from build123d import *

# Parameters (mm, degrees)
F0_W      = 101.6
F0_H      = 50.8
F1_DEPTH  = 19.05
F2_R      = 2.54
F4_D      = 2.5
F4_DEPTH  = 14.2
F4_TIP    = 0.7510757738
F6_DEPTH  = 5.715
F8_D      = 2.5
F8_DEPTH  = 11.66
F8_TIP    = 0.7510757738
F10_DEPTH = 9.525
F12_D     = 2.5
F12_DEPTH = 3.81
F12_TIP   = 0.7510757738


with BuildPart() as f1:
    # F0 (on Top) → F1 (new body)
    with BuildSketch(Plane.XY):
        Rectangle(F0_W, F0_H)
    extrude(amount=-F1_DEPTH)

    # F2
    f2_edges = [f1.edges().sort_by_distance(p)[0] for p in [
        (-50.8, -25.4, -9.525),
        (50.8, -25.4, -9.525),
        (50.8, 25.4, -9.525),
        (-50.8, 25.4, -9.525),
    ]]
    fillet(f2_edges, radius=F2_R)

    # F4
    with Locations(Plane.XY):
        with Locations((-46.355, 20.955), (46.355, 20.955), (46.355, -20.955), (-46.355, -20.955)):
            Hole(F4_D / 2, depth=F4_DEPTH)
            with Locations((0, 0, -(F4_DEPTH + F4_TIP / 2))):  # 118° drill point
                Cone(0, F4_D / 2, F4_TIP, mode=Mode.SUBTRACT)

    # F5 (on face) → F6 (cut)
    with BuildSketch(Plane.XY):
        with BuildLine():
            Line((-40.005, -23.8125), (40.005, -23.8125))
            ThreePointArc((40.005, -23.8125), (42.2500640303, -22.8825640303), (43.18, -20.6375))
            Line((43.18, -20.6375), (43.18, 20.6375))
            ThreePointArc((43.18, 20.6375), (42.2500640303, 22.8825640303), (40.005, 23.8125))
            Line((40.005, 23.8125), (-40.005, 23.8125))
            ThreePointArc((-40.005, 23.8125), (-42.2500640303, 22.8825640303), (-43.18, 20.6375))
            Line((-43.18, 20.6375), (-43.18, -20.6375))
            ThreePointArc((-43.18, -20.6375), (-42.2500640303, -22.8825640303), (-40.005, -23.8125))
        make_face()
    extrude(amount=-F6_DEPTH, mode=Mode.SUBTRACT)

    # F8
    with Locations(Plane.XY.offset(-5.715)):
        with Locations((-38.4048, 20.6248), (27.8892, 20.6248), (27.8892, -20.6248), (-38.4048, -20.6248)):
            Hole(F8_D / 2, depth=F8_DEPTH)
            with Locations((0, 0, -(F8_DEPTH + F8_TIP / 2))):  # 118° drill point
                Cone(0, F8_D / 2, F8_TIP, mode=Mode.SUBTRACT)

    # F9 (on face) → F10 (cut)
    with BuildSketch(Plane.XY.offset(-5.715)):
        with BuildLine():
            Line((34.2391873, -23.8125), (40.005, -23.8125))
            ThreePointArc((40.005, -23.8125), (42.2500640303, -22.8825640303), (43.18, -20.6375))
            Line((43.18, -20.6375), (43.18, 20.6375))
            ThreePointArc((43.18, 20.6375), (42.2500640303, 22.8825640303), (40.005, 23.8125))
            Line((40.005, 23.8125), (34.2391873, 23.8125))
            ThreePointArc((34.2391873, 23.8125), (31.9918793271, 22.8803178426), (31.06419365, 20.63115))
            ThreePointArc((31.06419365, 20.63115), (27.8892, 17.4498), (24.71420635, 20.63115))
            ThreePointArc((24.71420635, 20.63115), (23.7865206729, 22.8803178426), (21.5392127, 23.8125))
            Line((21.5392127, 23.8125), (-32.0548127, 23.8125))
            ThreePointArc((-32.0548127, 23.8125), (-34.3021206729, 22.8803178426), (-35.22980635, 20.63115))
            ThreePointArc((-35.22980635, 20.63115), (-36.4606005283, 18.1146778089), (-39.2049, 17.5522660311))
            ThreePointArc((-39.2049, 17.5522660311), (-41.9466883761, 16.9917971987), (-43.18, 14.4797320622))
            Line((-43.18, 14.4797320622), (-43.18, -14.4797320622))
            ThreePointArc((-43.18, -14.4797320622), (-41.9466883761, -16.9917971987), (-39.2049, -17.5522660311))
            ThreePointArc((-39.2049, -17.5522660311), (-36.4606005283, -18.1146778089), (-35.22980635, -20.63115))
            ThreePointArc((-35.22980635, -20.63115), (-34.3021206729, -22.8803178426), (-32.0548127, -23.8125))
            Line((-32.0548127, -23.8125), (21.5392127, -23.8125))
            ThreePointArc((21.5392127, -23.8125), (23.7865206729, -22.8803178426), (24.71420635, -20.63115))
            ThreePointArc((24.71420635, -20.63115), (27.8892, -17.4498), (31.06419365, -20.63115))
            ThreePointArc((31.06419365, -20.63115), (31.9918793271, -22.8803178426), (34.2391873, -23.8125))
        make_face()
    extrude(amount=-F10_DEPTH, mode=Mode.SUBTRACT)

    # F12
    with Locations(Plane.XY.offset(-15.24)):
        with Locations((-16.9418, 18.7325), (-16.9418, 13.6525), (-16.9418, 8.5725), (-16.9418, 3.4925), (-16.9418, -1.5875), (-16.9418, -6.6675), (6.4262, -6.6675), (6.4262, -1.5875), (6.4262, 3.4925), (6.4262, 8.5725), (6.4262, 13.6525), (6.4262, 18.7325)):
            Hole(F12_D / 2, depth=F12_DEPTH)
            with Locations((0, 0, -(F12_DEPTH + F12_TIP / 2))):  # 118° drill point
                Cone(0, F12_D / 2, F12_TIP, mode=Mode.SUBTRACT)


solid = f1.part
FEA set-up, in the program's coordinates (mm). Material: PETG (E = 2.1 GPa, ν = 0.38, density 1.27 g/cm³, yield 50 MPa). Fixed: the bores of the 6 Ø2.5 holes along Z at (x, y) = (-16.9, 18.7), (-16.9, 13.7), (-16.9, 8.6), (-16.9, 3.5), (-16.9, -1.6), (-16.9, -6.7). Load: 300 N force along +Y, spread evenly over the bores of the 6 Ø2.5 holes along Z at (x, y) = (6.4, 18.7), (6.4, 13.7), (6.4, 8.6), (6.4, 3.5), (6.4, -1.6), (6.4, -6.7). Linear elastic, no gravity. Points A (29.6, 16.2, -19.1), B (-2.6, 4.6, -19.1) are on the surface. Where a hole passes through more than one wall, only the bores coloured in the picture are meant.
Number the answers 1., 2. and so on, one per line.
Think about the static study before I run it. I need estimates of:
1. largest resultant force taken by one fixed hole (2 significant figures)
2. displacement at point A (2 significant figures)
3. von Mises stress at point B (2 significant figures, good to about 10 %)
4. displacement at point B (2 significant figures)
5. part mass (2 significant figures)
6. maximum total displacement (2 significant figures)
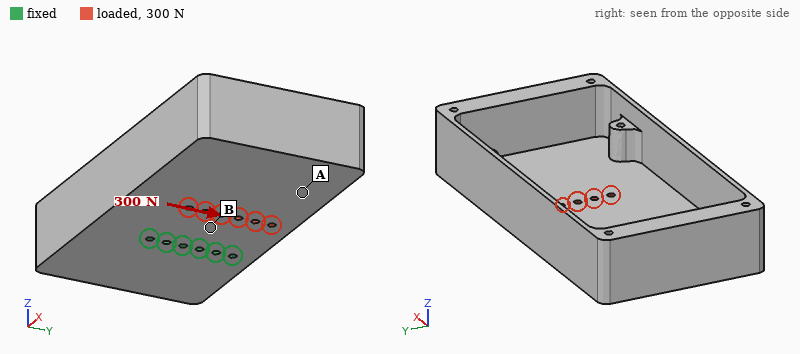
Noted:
1. 230 N
2. 0.16 mm
3. 4.4 MPa
4. 0.057 mm
5. 47 g
6. 0.23 mm
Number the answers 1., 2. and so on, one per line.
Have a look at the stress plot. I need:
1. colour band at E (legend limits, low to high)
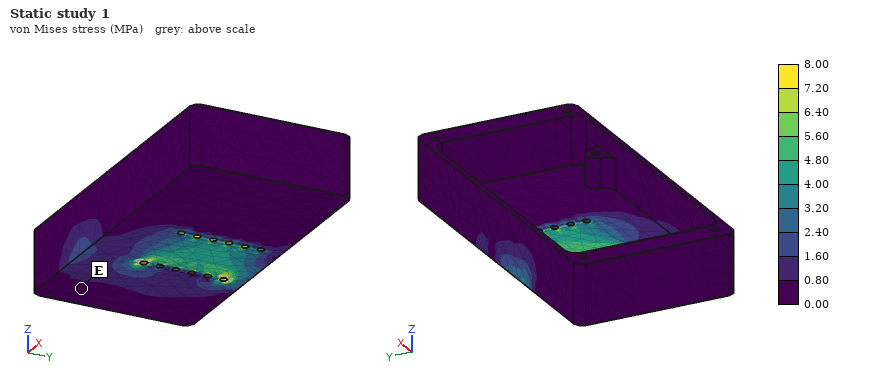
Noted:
1. 0.00 to 0.80 MPa
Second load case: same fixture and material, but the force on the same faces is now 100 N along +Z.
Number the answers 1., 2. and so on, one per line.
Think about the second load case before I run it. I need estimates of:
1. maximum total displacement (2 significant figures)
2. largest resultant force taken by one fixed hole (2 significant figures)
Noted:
1. 1.3 mm
2. 42 N
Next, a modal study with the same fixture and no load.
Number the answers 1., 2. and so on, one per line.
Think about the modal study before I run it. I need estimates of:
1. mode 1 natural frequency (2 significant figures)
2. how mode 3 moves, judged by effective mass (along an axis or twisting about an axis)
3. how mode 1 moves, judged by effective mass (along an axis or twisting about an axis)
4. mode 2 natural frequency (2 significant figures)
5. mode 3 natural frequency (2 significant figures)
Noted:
1. 190 Hz
2. along Z
3. along Z
4. 450 Hz
5. 650 Hz
